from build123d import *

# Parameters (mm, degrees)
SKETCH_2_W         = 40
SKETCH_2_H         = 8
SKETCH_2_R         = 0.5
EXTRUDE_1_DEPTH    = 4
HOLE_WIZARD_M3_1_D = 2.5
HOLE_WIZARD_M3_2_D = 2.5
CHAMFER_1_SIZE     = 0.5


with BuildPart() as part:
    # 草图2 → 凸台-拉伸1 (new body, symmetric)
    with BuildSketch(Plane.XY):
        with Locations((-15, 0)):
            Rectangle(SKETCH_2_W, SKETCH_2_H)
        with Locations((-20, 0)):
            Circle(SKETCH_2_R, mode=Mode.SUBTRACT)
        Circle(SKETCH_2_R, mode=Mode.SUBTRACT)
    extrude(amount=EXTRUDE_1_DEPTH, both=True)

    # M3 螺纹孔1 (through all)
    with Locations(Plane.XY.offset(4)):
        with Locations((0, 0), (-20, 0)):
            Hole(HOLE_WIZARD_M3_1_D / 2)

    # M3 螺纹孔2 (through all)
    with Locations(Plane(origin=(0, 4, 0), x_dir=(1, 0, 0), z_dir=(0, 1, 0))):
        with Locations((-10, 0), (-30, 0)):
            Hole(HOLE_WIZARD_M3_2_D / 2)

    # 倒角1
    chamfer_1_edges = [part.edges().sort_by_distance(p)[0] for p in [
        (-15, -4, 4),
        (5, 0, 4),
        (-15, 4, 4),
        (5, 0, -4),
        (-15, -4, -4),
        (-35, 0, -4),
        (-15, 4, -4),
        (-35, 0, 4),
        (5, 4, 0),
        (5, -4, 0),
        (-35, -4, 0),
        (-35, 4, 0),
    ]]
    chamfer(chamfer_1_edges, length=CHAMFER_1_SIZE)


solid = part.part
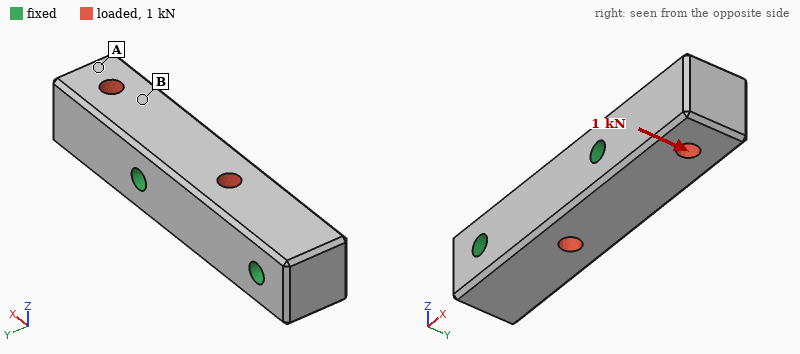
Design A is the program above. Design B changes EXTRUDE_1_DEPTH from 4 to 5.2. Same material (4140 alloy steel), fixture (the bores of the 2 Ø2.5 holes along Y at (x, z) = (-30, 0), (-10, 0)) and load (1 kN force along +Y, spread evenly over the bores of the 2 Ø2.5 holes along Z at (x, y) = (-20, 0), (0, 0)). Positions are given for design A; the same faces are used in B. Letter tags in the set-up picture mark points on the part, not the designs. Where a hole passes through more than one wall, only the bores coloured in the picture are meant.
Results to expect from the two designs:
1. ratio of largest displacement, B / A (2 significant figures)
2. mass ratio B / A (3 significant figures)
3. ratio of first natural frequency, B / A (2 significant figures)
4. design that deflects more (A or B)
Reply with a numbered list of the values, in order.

1. 0.83
2. 1.31
3. 1.1
4. A
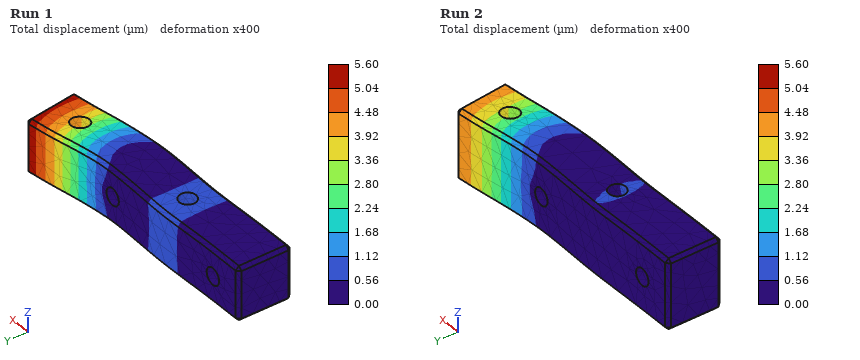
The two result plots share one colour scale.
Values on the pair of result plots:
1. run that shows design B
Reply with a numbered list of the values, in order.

1. Run 2
